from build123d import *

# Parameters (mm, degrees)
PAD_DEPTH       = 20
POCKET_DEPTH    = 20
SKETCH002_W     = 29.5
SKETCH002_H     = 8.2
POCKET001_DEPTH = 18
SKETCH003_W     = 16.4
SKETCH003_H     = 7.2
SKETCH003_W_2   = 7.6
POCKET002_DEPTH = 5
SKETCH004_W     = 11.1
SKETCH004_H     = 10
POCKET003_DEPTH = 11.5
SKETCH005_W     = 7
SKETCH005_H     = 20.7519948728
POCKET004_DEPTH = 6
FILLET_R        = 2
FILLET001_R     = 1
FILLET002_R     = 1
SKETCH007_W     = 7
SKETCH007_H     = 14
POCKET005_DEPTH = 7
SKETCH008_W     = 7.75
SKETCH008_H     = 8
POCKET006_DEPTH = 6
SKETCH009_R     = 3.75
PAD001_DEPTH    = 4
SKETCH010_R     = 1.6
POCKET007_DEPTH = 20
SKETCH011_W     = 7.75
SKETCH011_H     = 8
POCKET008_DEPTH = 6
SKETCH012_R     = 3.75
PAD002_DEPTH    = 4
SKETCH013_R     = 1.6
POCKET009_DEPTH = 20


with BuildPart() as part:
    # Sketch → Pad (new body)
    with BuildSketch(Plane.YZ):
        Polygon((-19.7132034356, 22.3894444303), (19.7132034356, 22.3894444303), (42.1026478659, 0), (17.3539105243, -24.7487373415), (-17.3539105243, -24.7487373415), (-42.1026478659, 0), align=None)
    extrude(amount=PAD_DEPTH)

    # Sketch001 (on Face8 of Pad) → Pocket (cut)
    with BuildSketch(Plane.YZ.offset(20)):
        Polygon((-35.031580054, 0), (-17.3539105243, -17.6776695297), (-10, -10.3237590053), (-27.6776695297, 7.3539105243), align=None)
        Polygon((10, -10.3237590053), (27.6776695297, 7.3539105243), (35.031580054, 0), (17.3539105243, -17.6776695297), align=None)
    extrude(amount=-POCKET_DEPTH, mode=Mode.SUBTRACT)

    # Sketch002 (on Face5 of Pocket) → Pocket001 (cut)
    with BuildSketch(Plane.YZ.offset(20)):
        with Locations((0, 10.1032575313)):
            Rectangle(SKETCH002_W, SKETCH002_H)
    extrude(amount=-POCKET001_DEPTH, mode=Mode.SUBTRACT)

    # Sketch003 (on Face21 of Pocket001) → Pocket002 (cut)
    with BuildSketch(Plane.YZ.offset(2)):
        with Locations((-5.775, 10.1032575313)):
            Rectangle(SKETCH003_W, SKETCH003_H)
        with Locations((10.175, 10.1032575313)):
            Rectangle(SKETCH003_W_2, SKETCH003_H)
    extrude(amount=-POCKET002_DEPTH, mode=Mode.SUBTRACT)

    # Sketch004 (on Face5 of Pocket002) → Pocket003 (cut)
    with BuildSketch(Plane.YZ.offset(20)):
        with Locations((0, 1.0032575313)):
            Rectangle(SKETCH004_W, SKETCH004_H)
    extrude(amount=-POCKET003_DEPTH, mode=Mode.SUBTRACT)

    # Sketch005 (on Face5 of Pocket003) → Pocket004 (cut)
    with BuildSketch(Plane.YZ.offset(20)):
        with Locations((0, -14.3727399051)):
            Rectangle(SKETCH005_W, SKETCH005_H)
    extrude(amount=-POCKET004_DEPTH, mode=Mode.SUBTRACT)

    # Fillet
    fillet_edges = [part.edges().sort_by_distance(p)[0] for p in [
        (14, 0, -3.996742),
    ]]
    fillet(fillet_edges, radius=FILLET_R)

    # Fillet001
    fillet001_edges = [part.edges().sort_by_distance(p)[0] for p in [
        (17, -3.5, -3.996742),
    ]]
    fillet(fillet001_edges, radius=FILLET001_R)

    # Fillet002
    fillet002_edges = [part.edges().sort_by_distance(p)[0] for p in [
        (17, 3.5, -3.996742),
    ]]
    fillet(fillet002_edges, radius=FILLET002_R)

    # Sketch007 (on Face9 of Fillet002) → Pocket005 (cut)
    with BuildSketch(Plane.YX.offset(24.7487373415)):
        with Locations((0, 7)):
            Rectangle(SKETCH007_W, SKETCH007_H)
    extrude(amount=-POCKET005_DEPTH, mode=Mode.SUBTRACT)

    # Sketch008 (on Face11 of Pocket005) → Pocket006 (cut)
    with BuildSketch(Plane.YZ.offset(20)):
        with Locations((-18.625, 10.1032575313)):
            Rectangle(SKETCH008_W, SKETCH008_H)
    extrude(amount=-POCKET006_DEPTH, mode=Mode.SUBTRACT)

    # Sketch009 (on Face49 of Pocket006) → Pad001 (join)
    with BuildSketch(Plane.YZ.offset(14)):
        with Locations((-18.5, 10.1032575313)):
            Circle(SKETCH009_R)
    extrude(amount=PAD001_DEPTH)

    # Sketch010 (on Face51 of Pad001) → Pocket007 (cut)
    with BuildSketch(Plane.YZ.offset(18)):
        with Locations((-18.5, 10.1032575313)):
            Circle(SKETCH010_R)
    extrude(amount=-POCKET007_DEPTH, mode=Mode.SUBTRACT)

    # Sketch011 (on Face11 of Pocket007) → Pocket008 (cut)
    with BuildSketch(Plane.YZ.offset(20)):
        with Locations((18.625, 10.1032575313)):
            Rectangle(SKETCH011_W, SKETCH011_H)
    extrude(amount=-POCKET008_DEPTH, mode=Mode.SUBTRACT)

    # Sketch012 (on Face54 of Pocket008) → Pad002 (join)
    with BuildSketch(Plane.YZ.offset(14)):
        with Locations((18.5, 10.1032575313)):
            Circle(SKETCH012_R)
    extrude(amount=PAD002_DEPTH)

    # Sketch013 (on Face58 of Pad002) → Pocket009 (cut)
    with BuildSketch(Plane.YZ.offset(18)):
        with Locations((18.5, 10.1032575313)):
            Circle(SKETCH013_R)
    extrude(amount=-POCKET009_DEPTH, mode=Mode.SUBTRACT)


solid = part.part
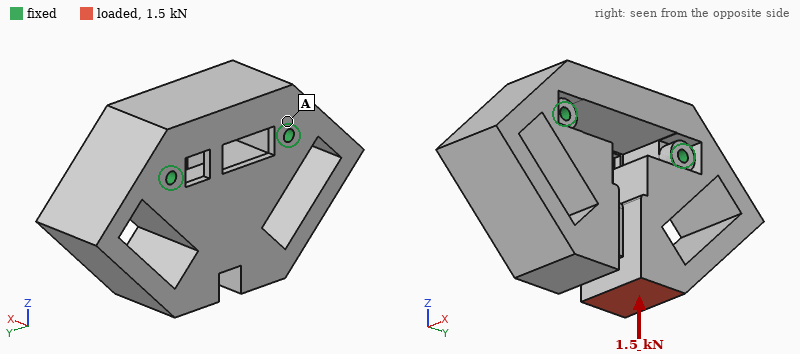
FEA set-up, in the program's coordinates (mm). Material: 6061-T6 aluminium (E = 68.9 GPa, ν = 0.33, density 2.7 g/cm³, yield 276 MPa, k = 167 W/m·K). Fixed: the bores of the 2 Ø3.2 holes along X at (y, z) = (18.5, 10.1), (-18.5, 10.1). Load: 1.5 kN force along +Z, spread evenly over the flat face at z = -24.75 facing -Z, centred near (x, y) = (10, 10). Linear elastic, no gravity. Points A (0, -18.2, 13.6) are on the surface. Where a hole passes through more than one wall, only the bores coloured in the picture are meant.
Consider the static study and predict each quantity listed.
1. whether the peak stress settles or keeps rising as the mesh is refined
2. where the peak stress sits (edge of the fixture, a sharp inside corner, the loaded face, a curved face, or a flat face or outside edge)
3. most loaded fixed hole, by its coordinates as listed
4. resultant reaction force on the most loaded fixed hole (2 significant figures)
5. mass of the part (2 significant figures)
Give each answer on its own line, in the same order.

keeps rising
a sharp inside corner
(18.5, 10.1)
1.2 kN
100 g
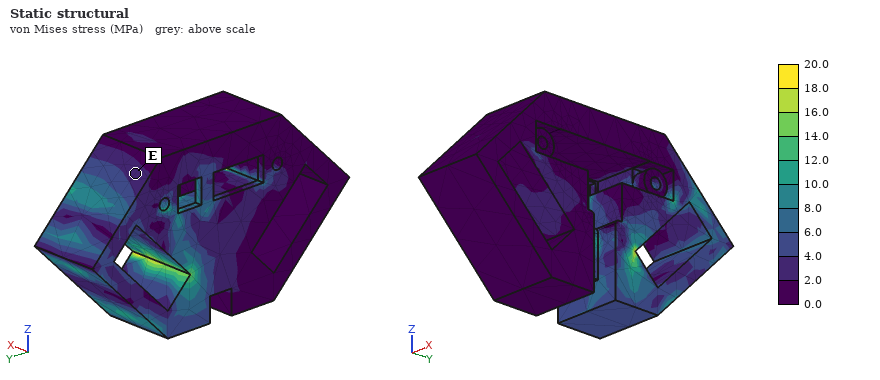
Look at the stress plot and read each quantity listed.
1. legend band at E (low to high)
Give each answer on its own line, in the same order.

2.0 to 4.0 MPa
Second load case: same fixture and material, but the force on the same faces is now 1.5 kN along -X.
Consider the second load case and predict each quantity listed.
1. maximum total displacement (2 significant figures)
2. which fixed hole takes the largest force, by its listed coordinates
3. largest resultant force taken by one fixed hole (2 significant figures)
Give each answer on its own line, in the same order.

82 µm
(18.5, 10.1)
1.1 kN
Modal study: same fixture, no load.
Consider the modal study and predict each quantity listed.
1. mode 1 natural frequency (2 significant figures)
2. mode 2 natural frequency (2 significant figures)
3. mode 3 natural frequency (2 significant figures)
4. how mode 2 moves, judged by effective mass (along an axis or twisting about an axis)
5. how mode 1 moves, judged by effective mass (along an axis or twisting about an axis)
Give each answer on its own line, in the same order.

5400 Hz
9400 Hz
10 kHz
along Y
along X
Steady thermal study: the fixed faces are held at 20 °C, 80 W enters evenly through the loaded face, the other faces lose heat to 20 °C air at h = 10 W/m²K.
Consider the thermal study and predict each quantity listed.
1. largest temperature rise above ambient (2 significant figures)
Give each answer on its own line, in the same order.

52 K
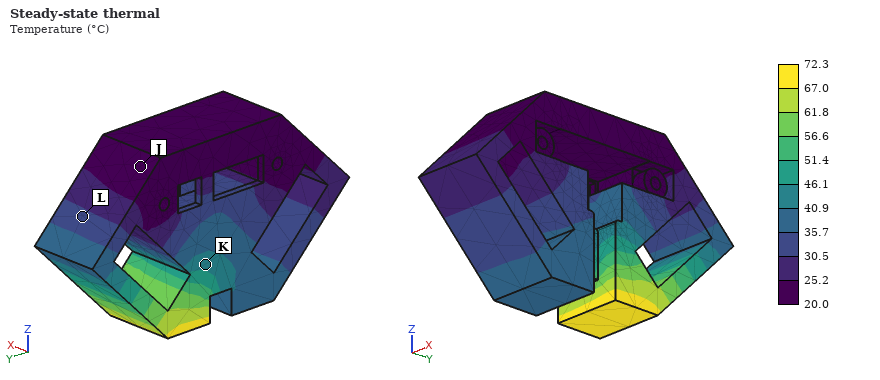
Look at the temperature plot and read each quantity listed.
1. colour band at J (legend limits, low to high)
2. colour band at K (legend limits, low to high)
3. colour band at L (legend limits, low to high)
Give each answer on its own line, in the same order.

20.0 to 25.2 °C
40.9 to 46.1 °C
30.5 to 35.7 °C
